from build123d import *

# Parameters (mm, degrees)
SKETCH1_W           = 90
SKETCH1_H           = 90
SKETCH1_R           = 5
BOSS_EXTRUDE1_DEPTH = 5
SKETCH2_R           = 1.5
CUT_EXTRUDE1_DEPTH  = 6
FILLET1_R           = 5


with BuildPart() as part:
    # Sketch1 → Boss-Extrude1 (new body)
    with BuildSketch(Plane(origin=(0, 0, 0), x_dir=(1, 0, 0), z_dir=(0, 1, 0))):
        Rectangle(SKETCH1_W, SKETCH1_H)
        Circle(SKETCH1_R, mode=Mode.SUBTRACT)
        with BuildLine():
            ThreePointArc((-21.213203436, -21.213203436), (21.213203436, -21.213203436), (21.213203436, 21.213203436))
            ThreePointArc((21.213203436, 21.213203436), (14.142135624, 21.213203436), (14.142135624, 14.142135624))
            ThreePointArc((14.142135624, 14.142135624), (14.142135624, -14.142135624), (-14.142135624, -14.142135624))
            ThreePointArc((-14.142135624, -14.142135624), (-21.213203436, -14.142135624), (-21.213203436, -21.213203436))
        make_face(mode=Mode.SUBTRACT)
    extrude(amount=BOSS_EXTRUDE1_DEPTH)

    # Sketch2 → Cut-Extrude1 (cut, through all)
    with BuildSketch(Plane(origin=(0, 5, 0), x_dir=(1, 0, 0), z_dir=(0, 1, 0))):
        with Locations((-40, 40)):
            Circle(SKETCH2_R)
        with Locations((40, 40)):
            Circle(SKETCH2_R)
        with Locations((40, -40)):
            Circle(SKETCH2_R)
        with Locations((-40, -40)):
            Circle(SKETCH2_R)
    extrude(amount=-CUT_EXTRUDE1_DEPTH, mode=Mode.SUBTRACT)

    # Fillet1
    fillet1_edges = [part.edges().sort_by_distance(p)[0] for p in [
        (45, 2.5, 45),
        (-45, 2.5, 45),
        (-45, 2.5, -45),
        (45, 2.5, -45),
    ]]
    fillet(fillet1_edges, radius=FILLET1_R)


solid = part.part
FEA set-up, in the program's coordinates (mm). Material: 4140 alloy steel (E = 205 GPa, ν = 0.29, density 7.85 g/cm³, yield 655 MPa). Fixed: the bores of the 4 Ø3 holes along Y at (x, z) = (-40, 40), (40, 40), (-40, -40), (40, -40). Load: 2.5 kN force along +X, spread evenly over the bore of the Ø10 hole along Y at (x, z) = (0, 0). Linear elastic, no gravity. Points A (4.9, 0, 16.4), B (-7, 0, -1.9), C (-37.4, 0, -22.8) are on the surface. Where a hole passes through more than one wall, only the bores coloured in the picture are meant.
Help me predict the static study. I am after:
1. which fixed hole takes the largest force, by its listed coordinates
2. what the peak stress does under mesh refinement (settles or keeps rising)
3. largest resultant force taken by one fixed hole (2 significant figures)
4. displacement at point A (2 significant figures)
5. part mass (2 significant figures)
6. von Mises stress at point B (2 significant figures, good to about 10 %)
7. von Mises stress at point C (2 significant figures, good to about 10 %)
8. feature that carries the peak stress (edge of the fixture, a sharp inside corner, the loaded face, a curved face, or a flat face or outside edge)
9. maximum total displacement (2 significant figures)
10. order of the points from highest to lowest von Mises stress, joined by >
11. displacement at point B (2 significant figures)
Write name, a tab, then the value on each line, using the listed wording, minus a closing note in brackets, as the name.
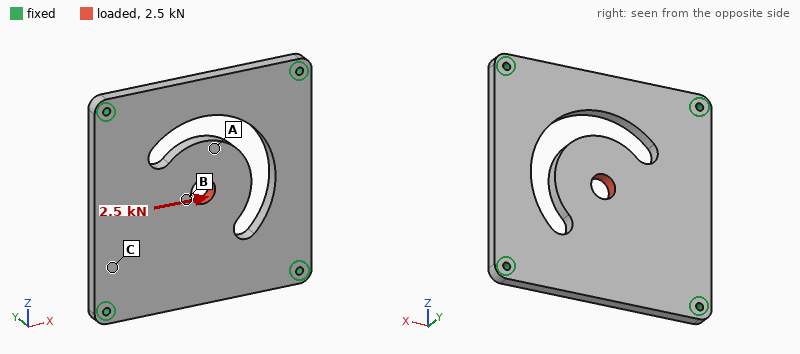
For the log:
which fixed hole takes the largest force, by its listed coordinates	(-40, -40)
what the peak stress does under mesh refinement	keeps rising
largest resultant force taken by one fixed hole	1.2 kN
displacement at point A	8.7 µm
part mass	280 g
von Mises stress at point B	15 MPa
von Mises stress at point C	9.1 MPa
feature that carries the peak stress	edge of the fixture
maximum total displacement	9.0 µm
order of the points from highest to lowest von Mises stress, joined by >	B > C > A
displacement at point B	5.8 µm
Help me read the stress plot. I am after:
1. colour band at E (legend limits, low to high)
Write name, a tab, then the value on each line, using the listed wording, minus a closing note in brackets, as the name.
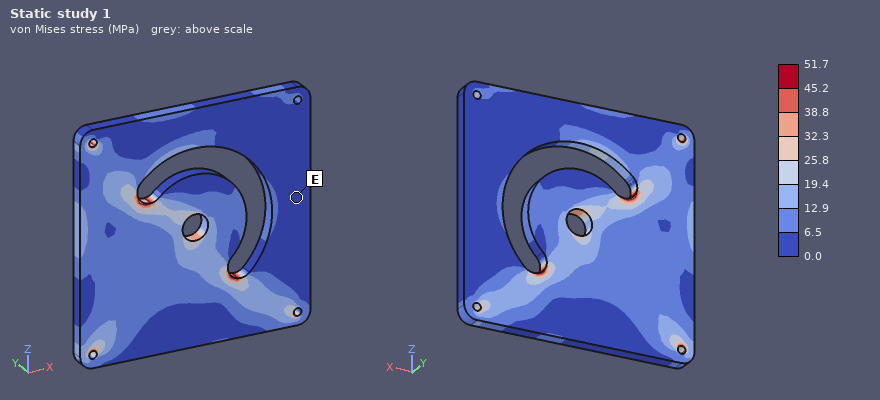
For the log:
colour band at E	0.0 to 6.5 MPa
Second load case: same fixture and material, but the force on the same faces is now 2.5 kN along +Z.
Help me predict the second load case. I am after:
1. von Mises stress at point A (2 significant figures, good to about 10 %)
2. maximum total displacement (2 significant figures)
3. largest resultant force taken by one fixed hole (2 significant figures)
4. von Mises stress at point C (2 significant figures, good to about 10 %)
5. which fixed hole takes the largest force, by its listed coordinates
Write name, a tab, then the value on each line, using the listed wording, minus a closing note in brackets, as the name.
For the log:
von Mises stress at point A	7.1 MPa
maximum total displacement	9.0 µm
largest resultant force taken by one fixed hole	1.2 kN
von Mises stress at point C	5.6 MPa
which fixed hole takes the largest force, by its listed coordinates	(-40, -40)
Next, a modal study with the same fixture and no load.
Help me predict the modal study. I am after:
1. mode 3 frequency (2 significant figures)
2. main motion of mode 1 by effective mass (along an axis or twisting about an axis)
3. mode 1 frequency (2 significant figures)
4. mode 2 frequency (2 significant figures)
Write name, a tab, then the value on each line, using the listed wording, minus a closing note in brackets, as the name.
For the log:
mode 3 frequency	4000 Hz
main motion of mode 1 by effective mass	along Y
mode 1 frequency	1800 Hz
mode 2 frequency	4000 Hz
